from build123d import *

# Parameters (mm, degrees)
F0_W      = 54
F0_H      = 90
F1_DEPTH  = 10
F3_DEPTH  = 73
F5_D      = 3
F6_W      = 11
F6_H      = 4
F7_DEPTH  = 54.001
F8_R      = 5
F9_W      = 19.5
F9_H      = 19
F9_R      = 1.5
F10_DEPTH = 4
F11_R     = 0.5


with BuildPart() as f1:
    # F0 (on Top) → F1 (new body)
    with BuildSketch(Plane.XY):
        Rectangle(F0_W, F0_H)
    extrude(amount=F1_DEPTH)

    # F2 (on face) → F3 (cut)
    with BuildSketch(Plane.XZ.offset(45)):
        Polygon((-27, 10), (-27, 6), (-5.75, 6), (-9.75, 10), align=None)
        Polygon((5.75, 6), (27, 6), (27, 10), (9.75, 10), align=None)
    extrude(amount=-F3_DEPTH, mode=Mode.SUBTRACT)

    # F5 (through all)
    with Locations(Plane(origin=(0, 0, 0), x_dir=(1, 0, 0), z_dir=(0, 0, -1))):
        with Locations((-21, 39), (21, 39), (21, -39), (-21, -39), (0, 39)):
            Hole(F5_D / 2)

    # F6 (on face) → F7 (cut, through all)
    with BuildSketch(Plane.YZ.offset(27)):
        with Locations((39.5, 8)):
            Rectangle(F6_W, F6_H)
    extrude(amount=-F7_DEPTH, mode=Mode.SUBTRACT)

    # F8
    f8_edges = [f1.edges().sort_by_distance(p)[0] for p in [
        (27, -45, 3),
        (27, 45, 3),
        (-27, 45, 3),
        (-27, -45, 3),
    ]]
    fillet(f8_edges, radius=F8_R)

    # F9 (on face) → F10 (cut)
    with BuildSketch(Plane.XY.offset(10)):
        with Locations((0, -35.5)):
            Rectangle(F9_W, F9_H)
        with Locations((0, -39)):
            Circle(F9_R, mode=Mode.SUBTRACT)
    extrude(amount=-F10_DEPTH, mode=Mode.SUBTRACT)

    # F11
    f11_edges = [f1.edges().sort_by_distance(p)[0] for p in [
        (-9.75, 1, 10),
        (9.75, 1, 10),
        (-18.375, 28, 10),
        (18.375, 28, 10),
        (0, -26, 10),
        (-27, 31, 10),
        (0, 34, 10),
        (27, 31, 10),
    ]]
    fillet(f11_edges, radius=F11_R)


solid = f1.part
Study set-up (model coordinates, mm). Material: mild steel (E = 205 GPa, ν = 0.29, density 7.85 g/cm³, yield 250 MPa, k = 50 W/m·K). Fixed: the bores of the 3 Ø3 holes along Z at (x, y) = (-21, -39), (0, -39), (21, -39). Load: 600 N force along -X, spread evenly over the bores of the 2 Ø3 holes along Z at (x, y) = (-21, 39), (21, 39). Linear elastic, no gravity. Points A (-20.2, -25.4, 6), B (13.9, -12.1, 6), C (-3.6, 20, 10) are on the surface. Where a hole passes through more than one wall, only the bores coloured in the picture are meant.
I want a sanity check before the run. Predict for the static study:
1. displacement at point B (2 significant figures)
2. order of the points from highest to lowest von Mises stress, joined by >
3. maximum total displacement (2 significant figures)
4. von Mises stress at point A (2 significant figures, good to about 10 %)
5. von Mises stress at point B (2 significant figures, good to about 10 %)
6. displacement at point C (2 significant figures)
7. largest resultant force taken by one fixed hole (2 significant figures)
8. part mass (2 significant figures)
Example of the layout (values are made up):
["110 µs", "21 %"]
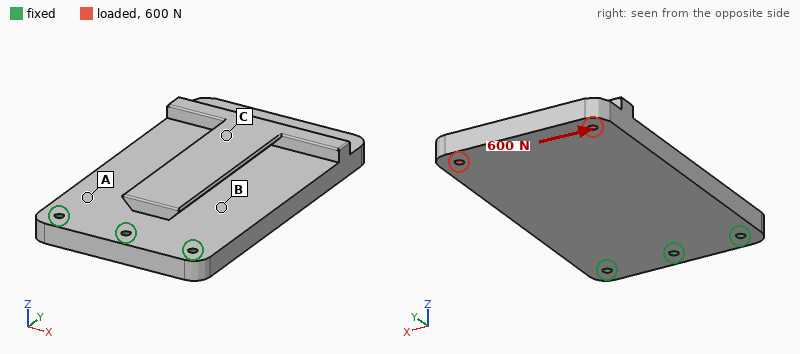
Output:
["2.1 µm", "A > B > C", "10 µm", "11 MPa", "6.1 MPa", "5.5 µm", "1.1 kN", "260 g"]
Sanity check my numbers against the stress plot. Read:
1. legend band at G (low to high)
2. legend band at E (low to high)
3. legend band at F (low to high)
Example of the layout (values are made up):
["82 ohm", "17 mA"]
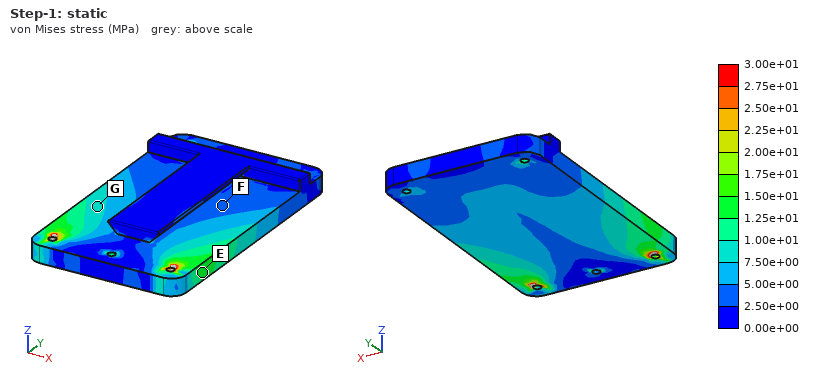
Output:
["7.50e+00 to 1.00e+01 MPa", "1.25e+01 to 1.50e+01 MPa", "2.50e+00 to 5.00e+00 MPa"]
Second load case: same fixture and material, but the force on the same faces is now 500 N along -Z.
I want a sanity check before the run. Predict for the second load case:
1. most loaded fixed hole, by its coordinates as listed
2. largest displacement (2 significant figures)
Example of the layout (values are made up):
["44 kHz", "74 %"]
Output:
["(0, -39)", "0.35 mm"]
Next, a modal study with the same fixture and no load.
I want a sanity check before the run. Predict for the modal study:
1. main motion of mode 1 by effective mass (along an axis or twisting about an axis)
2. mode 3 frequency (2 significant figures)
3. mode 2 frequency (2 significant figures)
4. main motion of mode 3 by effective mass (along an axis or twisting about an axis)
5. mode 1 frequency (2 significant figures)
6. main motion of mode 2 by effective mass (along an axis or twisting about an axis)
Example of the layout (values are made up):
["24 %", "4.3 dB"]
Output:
["along Z", "4400 Hz", "2600 Hz", "along X", "700 Hz", "twisting about Y"]
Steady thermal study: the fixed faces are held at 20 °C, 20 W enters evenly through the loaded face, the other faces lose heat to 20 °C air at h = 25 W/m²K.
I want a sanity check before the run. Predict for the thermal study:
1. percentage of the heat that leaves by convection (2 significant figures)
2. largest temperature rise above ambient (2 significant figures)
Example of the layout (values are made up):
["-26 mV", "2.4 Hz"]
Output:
["46 %", "71 K"]
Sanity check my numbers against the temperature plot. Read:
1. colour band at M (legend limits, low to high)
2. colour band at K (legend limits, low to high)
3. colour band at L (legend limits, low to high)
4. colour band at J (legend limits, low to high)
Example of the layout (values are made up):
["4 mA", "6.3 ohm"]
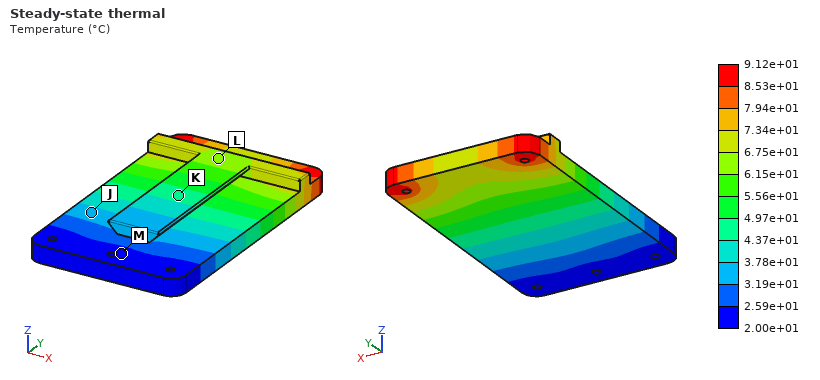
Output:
["2.00e+01 to 2.59e+01 °C", "4.37e+01 to 4.97e+01 °C", "6.15e+01 to 6.75e+01 °C", "3.19e+01 to 3.78e+01 °C"]
